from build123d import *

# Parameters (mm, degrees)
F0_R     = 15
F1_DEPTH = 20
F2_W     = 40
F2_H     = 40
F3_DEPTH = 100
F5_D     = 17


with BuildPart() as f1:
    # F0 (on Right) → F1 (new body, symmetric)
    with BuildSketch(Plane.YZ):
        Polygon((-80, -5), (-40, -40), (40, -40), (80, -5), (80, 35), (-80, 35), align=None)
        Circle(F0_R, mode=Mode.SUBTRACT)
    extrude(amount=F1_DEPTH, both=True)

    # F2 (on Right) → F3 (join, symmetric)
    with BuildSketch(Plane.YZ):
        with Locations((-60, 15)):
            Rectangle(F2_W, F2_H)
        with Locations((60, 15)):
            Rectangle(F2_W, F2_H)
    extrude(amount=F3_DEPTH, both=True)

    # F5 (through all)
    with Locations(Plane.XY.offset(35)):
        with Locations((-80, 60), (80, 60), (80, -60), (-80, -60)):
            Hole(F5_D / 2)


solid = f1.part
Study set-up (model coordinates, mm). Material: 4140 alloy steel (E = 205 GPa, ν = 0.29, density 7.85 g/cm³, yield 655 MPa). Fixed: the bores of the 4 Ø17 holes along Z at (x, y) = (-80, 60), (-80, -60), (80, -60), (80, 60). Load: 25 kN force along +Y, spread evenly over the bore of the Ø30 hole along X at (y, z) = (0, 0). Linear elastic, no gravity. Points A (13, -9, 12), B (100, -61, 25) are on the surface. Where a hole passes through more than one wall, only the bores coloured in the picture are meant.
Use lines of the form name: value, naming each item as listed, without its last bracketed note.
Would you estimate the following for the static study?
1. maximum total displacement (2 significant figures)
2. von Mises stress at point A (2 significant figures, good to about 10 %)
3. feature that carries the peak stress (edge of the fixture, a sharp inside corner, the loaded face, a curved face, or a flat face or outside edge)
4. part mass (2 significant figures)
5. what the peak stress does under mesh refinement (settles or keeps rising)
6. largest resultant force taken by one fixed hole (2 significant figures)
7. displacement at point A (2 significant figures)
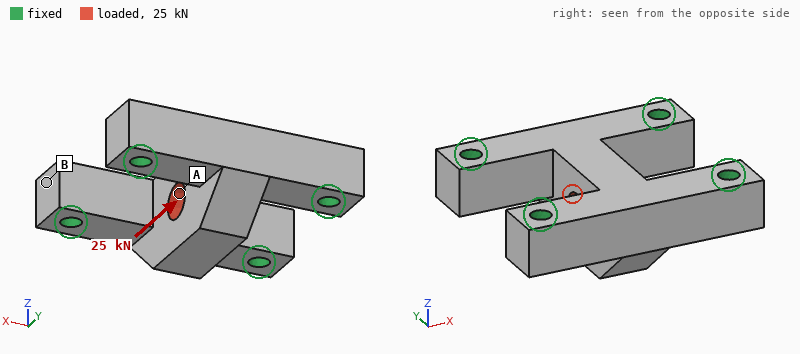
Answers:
maximum total displacement: 11 µm
von Mises stress at point A: 11 MPa
feature that carries the peak stress: edge of the fixture
part mass: 6.8 kg
what the peak stress does under mesh refinement: keeps rising
largest resultant force taken by one fixed hole: 6.5 kN
displacement at point A: 9.6 µm
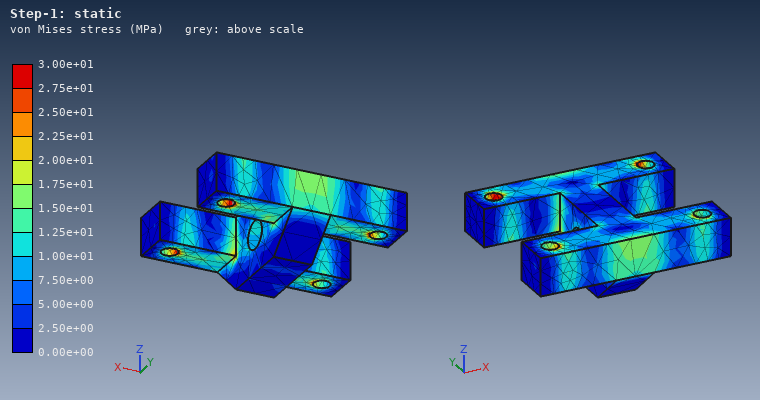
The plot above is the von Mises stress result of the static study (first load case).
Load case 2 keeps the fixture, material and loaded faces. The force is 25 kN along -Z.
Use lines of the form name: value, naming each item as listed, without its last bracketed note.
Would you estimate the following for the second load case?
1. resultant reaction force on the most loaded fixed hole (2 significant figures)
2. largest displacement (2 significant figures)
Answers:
resultant reaction force on the most loaded fixed hole: 6.3 kN
largest displacement: 13 µm
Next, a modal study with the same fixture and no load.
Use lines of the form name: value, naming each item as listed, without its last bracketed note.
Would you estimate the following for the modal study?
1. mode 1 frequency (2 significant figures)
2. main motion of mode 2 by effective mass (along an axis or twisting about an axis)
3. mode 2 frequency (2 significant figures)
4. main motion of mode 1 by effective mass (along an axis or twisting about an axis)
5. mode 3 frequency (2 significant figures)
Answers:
mode 1 frequency: 4100 Hz
main motion of mode 2 by effective mass: along Z
mode 2 frequency: 4500 Hz
main motion of mode 1 by effective mass: along Y
mode 3 frequency: 5900 Hz
